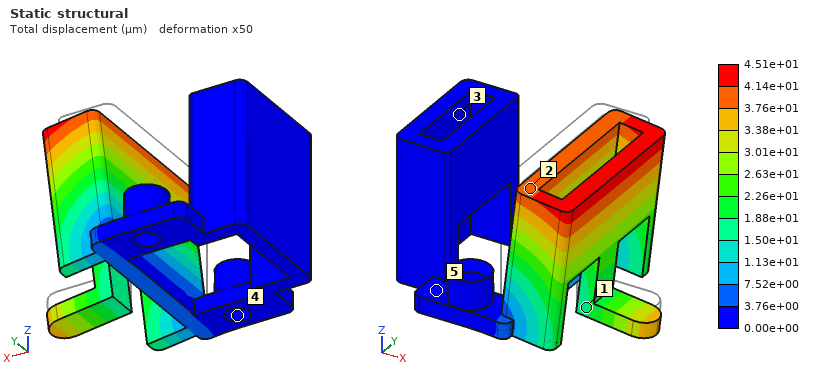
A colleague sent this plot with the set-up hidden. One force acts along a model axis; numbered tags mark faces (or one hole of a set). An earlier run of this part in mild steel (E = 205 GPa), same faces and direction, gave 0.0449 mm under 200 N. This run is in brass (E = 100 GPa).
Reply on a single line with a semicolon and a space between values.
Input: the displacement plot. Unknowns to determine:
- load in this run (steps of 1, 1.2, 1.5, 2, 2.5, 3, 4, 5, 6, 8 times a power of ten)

100 N
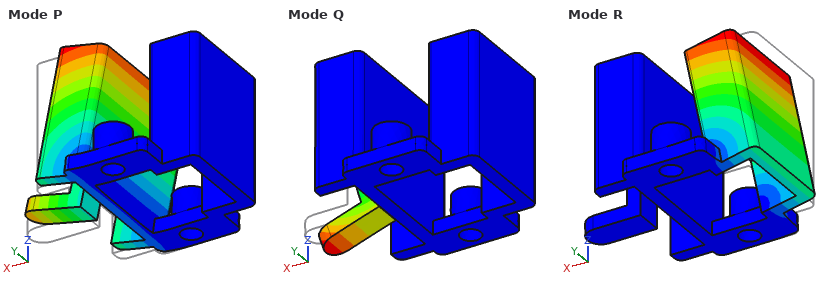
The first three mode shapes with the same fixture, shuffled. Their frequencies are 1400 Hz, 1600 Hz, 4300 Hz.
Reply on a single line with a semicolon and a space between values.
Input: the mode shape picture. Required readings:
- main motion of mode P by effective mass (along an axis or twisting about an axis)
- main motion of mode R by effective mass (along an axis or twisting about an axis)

along X; along X
